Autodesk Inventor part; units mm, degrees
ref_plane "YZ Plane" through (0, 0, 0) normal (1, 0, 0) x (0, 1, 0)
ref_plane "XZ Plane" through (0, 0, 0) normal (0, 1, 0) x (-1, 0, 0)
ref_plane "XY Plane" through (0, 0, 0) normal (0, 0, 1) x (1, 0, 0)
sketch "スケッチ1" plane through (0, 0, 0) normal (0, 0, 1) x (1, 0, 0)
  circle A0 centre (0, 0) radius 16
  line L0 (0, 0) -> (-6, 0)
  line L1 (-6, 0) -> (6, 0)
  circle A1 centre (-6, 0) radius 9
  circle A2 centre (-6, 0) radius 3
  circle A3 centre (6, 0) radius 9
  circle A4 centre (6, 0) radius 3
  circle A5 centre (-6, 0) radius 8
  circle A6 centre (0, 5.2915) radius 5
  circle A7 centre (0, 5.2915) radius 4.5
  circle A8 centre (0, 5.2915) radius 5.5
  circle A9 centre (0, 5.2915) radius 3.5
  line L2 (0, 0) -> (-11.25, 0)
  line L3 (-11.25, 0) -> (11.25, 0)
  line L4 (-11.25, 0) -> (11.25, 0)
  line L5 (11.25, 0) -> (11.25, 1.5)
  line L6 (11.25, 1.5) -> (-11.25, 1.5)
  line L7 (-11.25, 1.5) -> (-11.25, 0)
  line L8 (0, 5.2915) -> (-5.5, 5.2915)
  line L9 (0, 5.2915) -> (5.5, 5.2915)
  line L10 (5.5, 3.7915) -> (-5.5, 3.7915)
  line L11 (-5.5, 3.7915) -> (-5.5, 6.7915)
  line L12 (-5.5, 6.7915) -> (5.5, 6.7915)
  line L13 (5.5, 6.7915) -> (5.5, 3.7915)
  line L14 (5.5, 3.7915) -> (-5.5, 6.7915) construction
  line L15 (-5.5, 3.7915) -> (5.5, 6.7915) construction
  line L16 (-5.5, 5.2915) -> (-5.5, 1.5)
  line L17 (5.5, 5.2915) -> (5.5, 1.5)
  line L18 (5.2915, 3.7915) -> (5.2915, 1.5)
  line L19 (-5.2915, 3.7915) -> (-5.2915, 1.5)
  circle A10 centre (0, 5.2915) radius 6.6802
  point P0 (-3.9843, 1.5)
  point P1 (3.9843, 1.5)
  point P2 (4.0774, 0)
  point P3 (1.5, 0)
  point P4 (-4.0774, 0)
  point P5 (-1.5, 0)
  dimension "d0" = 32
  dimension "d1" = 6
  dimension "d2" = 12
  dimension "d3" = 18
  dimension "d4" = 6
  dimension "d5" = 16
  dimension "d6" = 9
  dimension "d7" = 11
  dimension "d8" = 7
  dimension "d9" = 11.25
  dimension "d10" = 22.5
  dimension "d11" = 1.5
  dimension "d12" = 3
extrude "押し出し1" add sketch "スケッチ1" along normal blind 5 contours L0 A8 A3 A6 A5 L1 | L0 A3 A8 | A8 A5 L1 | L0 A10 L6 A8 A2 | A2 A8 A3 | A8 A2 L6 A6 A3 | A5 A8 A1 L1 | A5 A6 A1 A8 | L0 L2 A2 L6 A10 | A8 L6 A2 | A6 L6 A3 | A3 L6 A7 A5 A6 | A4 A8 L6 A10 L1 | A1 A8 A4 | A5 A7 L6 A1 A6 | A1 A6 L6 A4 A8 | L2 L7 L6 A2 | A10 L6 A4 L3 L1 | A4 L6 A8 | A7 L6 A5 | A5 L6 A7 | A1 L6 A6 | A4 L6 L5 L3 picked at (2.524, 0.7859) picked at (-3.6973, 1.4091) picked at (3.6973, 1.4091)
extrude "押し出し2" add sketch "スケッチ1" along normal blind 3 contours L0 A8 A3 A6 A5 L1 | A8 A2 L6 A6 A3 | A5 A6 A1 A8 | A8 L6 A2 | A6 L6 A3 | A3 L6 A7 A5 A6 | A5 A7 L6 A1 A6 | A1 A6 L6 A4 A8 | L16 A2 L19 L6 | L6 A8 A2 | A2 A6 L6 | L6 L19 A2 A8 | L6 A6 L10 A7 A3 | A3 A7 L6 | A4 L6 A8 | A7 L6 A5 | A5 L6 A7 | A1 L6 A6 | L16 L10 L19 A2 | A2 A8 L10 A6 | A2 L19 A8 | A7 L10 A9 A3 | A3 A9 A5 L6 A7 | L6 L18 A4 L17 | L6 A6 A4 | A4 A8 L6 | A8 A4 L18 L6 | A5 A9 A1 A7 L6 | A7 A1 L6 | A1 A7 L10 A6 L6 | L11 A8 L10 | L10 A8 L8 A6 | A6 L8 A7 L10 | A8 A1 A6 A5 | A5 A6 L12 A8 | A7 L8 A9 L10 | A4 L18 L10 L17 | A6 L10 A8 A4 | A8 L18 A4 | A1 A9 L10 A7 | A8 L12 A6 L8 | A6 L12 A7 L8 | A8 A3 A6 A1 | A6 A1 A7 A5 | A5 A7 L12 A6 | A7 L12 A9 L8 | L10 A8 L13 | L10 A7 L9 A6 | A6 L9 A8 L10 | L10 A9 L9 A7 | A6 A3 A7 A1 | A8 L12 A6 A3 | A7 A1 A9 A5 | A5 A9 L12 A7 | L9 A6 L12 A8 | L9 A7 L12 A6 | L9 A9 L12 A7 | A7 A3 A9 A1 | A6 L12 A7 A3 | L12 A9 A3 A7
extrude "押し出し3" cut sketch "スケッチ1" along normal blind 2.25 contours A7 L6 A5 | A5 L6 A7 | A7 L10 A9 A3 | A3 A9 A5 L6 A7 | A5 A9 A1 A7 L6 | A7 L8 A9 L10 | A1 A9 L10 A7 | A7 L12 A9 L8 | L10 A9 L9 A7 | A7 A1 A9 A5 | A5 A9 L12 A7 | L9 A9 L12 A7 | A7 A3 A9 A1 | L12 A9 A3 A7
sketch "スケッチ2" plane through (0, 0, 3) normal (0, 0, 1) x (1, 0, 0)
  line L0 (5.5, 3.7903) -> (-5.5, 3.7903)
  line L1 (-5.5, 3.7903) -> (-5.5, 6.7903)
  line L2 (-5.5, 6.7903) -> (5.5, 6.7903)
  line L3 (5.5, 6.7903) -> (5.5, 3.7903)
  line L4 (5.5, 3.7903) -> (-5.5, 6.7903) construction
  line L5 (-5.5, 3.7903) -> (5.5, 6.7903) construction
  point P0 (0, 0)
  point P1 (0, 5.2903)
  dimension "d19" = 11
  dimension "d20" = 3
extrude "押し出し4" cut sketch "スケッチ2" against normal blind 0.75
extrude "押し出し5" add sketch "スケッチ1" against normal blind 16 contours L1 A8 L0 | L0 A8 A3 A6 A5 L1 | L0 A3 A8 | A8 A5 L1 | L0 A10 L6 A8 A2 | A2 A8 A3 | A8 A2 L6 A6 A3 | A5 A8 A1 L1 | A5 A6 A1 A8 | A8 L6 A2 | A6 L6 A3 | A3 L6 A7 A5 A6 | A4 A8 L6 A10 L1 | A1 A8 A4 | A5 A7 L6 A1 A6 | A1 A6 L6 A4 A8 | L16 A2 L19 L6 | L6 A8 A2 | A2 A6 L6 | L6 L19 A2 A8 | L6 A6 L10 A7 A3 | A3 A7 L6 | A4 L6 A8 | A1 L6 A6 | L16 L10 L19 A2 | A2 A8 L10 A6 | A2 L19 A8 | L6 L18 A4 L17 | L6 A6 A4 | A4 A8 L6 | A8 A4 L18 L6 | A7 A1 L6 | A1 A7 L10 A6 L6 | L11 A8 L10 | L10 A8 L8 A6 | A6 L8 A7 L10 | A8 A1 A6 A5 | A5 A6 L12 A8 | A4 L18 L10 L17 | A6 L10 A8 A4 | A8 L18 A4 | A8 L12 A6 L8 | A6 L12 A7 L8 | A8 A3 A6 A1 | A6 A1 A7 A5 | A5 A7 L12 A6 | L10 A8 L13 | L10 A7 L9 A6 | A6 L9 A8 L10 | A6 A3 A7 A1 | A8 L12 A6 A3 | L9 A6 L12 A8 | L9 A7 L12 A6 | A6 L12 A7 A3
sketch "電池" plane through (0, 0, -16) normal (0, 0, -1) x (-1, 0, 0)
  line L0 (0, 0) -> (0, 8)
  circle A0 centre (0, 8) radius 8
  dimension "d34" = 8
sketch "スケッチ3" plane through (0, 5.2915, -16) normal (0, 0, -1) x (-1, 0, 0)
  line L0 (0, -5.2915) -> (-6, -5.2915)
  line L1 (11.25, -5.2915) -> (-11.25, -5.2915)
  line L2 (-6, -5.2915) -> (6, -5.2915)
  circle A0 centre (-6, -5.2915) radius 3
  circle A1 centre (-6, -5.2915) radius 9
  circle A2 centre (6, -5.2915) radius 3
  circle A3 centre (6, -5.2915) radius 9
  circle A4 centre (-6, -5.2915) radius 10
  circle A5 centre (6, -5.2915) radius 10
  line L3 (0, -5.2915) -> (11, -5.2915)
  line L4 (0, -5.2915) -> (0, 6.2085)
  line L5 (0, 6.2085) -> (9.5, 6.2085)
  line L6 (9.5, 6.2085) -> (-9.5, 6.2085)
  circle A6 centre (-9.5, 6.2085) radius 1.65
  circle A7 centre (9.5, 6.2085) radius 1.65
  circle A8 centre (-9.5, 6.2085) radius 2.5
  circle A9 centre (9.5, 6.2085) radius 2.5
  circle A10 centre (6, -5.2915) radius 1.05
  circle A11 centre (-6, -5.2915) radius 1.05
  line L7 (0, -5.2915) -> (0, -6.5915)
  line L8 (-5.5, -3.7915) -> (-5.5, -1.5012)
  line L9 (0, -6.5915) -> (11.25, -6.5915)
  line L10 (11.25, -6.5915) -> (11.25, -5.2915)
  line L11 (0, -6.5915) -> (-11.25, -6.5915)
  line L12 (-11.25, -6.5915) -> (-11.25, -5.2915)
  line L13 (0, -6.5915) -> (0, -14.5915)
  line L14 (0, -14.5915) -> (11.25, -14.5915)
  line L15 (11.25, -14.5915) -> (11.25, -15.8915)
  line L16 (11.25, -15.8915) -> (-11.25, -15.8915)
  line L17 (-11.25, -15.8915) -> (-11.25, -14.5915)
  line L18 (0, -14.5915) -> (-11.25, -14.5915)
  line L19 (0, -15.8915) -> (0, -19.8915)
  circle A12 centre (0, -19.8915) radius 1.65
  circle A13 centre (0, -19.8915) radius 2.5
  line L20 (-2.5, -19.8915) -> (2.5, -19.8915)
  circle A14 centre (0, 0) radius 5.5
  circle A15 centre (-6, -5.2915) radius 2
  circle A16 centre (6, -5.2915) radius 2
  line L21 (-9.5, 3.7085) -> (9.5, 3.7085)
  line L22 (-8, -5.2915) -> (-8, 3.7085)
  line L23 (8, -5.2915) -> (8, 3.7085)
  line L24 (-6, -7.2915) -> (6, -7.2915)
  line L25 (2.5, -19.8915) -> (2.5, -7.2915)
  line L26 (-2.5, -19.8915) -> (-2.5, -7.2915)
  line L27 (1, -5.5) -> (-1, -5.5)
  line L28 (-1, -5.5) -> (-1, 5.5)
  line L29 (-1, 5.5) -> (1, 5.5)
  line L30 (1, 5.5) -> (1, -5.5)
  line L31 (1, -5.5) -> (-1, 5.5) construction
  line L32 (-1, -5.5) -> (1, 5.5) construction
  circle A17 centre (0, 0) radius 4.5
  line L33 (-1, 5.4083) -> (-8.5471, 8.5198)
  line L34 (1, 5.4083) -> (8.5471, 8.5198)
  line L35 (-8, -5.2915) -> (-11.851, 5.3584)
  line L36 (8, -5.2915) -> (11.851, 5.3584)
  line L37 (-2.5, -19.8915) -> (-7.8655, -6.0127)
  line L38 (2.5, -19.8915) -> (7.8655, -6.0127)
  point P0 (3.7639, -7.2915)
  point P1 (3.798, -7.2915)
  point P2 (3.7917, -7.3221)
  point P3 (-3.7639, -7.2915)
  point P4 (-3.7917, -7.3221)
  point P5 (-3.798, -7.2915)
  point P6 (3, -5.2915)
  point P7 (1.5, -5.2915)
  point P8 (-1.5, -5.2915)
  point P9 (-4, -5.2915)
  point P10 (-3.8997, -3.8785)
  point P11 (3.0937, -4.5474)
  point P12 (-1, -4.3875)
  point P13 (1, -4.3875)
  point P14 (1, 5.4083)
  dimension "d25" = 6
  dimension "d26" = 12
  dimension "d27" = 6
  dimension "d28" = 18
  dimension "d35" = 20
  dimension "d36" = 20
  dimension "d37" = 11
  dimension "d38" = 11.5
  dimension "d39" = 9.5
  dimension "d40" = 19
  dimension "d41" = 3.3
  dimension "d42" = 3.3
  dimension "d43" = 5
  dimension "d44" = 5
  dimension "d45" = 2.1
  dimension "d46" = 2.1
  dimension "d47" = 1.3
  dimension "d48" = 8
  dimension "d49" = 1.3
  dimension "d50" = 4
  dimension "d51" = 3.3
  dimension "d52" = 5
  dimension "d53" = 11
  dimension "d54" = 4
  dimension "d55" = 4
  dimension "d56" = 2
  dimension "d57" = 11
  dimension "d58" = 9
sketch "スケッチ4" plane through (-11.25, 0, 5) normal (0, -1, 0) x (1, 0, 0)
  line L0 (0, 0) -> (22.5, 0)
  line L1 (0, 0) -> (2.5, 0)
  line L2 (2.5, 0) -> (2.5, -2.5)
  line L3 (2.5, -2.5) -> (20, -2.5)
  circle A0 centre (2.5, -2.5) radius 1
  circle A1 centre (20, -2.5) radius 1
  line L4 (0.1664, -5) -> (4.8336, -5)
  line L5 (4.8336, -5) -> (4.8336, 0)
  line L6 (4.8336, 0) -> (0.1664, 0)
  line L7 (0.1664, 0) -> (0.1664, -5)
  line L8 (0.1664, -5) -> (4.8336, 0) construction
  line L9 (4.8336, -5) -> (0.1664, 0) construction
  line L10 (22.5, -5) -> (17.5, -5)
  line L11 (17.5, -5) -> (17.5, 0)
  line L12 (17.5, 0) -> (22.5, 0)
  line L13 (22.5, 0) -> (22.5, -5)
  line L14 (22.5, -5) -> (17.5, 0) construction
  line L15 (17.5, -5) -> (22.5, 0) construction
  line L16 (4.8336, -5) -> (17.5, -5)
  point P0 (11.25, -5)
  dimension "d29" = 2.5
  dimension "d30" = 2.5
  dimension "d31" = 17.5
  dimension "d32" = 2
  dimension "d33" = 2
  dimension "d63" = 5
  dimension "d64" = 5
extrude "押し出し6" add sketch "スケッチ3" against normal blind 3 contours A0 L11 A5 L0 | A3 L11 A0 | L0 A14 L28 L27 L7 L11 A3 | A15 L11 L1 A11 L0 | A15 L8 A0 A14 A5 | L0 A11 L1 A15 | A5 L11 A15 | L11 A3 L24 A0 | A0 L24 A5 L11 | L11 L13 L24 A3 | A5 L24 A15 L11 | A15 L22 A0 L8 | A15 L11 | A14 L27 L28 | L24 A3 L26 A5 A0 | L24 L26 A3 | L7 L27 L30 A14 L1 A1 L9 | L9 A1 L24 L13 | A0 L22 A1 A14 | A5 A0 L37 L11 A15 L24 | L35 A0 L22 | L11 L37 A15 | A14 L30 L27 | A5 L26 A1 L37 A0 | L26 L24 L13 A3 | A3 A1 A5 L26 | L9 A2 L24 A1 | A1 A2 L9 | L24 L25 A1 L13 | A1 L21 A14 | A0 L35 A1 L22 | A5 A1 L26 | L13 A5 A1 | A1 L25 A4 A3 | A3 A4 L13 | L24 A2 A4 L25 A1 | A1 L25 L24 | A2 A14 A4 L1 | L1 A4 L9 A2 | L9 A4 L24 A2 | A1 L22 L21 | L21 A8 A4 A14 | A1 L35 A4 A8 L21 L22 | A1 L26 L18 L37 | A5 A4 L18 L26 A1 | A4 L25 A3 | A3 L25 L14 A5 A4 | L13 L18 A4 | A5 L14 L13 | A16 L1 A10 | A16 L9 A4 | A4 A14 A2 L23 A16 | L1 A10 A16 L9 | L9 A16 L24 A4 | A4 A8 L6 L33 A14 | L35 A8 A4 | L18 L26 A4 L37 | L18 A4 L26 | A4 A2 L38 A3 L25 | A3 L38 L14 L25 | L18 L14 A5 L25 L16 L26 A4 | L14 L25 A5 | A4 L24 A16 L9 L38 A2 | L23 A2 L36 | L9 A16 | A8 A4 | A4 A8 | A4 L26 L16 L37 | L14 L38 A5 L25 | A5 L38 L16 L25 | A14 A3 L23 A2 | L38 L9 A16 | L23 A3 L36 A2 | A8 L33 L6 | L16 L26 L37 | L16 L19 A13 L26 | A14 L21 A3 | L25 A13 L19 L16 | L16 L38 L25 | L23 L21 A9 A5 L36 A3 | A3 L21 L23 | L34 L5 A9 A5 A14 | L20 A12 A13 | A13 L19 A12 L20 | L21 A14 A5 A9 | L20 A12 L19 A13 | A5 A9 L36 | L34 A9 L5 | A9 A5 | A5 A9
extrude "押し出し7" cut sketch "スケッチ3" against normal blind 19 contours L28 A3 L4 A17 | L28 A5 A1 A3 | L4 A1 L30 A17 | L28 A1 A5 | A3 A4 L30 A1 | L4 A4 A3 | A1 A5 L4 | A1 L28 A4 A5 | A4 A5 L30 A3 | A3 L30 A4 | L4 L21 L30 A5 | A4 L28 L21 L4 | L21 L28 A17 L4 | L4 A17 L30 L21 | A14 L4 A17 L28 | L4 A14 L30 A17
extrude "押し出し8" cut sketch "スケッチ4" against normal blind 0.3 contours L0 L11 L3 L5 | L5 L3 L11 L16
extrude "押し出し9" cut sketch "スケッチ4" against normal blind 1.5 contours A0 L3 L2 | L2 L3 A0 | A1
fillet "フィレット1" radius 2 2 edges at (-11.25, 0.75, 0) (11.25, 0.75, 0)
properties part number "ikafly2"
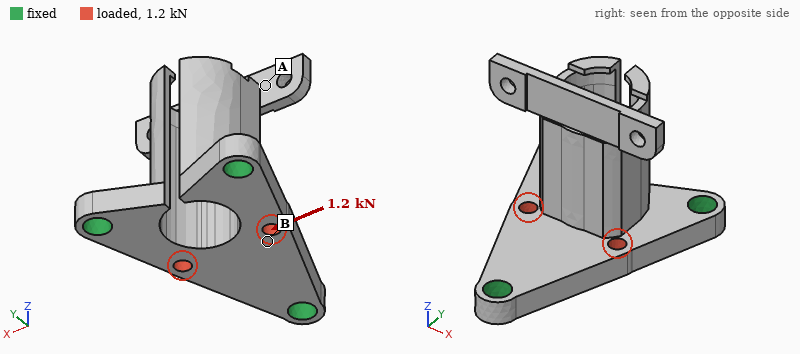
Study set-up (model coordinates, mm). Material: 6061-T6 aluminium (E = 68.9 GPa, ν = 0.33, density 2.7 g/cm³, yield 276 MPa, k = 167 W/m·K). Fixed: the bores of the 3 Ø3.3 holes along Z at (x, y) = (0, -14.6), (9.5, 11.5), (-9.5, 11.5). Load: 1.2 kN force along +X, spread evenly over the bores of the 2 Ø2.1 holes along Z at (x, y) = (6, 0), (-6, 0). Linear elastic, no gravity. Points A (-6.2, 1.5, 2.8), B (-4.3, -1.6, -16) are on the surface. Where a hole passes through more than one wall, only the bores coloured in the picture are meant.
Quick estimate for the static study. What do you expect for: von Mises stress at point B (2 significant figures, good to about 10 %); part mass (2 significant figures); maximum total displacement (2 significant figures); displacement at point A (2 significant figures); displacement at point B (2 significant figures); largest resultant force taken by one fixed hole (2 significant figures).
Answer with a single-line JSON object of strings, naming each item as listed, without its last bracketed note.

{"von Mises stress at point B": "35 MPa", "part mass": "4.6 g", "maximum total displacement": "27 µm", "displacement at point A": "13 µm", "displacement at point B": "24 µm", "largest resultant force taken by one fixed hole": "430 N"}
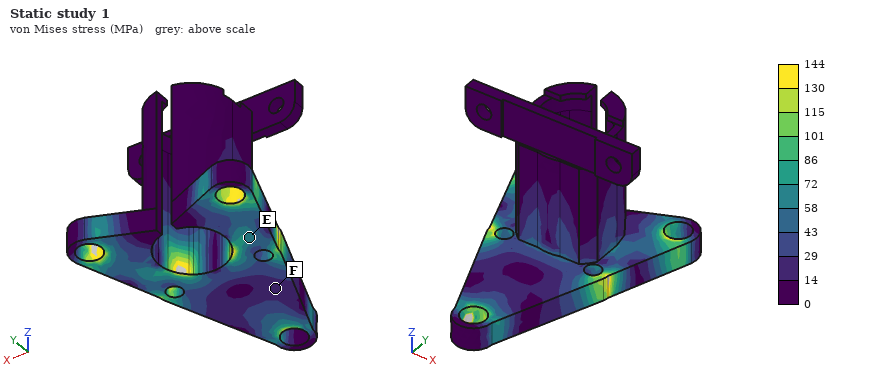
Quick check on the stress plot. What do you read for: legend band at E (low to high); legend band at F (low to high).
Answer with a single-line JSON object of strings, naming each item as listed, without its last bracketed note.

{"legend band at E": "58 to 72 MPa", "legend band at F": "14 to 29 MPa"}
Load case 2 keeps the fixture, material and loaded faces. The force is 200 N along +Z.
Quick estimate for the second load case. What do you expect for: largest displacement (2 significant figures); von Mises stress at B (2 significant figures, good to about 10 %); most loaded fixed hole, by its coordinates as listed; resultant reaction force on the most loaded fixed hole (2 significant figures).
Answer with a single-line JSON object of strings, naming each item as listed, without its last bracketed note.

{"largest displacement": "22 µm", "von Mises stress at B": "29 MPa", "most loaded fixed hole, by its coordinates as listed": "(0, -14.6)", "resultant reaction force on the most loaded fixed hole": "76 N"}
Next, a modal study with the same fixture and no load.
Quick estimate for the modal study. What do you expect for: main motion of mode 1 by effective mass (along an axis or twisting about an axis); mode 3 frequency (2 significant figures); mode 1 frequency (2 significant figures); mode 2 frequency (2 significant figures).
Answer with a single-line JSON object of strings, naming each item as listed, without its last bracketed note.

{"main motion of mode 1 by effective mass": "along X", "mode 3 frequency": "11 kHz", "mode 1 frequency": "7700 Hz", "mode 2 frequency": "8400 Hz"}
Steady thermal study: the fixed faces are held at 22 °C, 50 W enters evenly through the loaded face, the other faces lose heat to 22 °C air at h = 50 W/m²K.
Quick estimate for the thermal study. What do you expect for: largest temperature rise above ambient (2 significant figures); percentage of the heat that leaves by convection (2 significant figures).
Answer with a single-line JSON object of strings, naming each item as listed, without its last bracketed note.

{"largest temperature rise above ambient": "57 K", "percentage of the heat that leaves by convection": "5.8 %"}
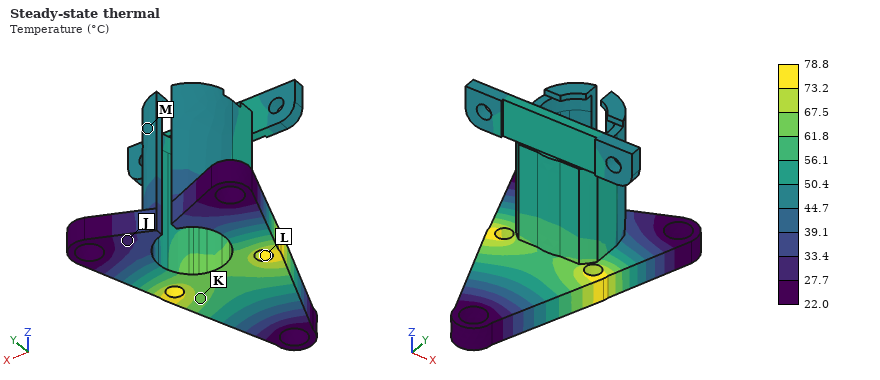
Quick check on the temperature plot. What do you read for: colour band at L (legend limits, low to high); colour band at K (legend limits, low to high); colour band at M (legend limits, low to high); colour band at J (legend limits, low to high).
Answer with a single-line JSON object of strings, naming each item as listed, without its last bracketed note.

{"colour band at L": "73.2 to 78.8 °C", "colour band at K": "61.8 to 67.5 °C", "colour band at M": "44.7 to 50.4 °C", "colour band at J": "27.7 to 33.4 °C"}
